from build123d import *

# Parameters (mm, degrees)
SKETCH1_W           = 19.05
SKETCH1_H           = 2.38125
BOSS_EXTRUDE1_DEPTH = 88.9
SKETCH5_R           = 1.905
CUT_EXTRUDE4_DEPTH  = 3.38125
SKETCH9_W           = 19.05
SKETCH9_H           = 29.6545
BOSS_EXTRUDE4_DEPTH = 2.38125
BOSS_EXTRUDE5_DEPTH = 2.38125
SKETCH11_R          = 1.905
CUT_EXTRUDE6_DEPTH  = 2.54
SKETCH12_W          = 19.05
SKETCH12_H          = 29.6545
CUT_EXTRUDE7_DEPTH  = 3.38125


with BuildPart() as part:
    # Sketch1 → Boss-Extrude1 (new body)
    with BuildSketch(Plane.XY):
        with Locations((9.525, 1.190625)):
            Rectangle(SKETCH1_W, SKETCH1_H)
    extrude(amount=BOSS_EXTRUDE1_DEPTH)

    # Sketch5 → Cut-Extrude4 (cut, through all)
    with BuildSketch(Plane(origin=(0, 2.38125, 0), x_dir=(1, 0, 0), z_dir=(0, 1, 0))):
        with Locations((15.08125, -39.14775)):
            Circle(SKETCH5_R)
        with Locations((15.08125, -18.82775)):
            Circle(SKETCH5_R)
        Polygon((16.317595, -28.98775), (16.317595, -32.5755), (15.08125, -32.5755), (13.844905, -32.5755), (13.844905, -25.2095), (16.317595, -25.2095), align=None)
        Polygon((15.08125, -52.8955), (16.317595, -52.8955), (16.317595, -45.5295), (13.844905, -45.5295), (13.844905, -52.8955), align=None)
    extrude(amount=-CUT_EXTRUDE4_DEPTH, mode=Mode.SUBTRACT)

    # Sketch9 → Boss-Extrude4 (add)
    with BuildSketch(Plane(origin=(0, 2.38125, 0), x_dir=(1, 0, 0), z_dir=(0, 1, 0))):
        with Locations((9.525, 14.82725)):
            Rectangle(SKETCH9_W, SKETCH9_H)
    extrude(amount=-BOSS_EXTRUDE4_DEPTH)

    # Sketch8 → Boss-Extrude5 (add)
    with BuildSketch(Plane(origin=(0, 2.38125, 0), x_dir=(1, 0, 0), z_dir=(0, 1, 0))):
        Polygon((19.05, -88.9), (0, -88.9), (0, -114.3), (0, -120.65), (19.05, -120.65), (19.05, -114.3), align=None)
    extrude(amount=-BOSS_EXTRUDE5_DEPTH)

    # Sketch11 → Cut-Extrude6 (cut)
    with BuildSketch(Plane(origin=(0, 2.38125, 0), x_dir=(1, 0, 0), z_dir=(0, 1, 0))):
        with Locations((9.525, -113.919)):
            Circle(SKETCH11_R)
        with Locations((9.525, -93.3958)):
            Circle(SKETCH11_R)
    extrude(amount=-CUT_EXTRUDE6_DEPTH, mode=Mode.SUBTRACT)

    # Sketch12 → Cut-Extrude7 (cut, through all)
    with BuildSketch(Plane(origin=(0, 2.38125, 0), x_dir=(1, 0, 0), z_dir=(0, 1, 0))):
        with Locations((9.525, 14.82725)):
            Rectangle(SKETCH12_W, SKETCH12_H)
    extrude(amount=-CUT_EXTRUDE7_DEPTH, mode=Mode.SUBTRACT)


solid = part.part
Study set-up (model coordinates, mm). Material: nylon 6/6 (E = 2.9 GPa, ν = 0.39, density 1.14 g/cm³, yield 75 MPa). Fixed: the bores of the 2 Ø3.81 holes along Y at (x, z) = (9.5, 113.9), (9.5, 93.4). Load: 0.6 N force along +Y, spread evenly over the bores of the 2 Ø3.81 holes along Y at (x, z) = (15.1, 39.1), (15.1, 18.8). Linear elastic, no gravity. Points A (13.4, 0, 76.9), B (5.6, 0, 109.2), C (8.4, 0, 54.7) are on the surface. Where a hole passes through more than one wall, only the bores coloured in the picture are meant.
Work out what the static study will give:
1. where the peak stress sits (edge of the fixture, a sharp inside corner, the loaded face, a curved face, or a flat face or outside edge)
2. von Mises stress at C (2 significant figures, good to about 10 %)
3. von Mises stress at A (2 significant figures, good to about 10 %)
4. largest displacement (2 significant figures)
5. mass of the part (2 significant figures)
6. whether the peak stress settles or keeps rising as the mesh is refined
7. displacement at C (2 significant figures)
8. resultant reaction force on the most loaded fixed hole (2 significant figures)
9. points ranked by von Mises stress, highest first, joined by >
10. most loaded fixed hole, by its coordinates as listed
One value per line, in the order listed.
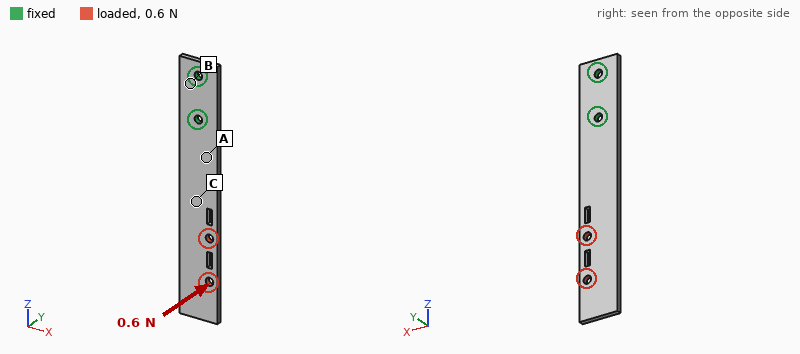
edge of the fixture
0.91 MPa
1.6 MPa
1.4 mm
6.0 g
keeps rising
0.35 mm
0.85 N
A > C > B
(9.5, 93.4)
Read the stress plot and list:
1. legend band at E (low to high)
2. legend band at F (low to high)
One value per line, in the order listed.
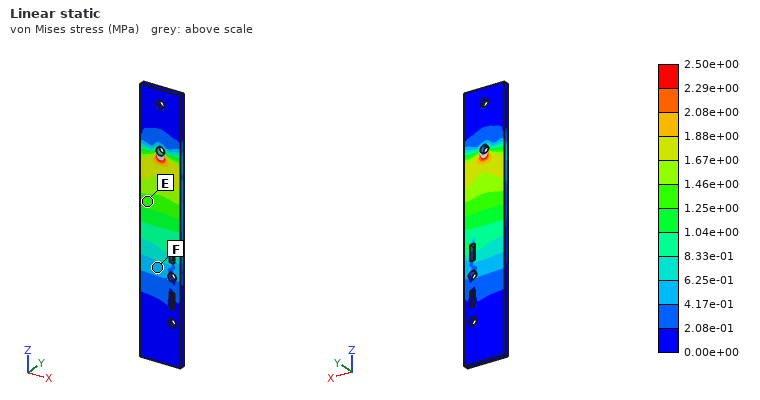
1.25e+00 to 1.46e+00 MPa
4.17e-01 to 6.25e-01 MPa
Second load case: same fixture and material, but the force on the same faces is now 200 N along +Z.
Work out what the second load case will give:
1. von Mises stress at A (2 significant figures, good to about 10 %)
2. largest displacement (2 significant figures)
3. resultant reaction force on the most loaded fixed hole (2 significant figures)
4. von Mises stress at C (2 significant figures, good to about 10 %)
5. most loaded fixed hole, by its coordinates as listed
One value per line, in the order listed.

7.7 MPa
1.5 mm
170 N
4.3 MPa
(9.5, 93.4)
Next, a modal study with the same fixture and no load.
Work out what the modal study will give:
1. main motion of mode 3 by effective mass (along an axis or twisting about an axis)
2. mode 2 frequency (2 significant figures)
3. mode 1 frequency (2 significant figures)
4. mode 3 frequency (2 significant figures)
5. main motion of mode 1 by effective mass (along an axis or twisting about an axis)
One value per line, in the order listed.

along X
440 Hz
73 Hz
470 Hz
along Y
